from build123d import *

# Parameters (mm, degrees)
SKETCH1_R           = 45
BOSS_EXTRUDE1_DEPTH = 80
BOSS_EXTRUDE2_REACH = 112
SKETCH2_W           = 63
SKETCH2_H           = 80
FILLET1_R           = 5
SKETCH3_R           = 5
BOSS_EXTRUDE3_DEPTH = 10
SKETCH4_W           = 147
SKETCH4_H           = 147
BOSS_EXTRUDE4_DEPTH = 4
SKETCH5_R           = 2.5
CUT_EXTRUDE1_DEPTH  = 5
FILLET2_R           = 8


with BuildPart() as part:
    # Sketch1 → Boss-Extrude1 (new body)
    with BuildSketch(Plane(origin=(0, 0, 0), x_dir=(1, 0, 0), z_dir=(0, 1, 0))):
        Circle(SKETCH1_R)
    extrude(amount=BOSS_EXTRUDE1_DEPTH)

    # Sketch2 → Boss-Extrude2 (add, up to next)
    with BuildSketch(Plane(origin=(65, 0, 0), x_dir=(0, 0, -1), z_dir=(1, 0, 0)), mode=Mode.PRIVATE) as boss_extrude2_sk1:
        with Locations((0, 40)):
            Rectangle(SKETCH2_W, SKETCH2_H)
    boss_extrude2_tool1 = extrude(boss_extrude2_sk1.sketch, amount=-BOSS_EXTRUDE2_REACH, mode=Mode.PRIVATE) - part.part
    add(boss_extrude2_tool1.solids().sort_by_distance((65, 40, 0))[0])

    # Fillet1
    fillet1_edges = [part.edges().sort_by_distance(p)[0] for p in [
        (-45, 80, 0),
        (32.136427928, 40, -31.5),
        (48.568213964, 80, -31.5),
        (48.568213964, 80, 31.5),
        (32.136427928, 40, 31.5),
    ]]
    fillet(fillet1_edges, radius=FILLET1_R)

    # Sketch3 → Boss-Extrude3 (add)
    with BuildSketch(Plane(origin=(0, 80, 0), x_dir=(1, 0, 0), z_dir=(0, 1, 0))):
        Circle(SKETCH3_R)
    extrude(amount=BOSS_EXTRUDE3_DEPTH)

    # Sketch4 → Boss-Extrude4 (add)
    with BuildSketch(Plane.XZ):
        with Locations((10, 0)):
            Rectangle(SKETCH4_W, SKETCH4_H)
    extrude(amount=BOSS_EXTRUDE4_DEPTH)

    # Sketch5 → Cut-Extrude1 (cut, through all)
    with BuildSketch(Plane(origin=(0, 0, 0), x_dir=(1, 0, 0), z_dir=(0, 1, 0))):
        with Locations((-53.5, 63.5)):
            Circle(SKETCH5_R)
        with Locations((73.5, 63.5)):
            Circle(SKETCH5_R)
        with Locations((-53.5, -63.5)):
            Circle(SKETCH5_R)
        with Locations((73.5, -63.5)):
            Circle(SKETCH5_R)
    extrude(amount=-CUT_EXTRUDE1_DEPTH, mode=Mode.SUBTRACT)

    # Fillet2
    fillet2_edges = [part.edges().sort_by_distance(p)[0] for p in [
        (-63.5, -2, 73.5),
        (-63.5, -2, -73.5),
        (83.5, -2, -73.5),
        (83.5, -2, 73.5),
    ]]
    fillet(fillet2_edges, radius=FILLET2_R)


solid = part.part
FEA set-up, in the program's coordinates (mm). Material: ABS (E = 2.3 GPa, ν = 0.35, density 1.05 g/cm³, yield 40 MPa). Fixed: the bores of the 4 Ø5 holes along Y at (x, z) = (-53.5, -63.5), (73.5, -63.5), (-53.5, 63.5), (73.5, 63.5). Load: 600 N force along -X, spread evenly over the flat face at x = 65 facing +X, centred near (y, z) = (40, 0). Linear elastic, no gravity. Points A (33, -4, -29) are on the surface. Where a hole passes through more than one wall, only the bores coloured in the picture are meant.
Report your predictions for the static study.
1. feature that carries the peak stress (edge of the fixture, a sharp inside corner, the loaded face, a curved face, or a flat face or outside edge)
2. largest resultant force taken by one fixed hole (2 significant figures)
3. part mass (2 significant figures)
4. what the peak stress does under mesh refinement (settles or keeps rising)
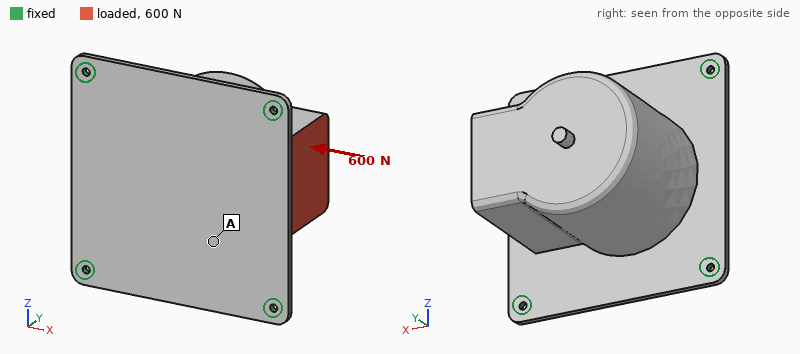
edge of the fixture
210 N
750 g
keeps rising
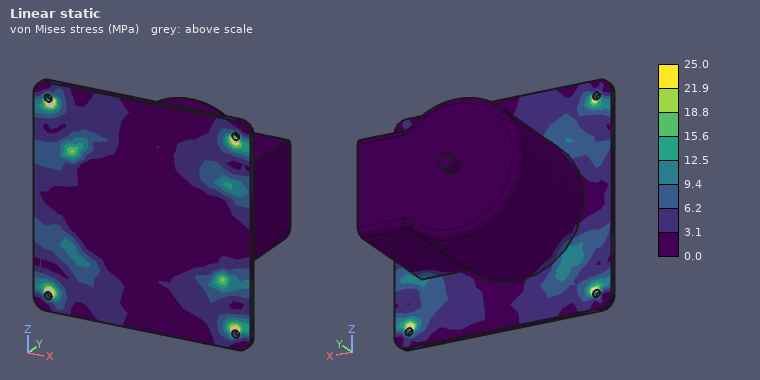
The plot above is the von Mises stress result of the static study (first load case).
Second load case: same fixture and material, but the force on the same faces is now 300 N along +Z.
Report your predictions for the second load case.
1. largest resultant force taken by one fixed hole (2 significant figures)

130 N
